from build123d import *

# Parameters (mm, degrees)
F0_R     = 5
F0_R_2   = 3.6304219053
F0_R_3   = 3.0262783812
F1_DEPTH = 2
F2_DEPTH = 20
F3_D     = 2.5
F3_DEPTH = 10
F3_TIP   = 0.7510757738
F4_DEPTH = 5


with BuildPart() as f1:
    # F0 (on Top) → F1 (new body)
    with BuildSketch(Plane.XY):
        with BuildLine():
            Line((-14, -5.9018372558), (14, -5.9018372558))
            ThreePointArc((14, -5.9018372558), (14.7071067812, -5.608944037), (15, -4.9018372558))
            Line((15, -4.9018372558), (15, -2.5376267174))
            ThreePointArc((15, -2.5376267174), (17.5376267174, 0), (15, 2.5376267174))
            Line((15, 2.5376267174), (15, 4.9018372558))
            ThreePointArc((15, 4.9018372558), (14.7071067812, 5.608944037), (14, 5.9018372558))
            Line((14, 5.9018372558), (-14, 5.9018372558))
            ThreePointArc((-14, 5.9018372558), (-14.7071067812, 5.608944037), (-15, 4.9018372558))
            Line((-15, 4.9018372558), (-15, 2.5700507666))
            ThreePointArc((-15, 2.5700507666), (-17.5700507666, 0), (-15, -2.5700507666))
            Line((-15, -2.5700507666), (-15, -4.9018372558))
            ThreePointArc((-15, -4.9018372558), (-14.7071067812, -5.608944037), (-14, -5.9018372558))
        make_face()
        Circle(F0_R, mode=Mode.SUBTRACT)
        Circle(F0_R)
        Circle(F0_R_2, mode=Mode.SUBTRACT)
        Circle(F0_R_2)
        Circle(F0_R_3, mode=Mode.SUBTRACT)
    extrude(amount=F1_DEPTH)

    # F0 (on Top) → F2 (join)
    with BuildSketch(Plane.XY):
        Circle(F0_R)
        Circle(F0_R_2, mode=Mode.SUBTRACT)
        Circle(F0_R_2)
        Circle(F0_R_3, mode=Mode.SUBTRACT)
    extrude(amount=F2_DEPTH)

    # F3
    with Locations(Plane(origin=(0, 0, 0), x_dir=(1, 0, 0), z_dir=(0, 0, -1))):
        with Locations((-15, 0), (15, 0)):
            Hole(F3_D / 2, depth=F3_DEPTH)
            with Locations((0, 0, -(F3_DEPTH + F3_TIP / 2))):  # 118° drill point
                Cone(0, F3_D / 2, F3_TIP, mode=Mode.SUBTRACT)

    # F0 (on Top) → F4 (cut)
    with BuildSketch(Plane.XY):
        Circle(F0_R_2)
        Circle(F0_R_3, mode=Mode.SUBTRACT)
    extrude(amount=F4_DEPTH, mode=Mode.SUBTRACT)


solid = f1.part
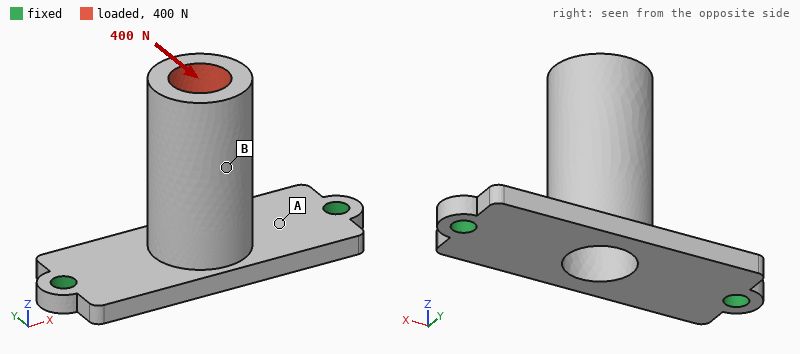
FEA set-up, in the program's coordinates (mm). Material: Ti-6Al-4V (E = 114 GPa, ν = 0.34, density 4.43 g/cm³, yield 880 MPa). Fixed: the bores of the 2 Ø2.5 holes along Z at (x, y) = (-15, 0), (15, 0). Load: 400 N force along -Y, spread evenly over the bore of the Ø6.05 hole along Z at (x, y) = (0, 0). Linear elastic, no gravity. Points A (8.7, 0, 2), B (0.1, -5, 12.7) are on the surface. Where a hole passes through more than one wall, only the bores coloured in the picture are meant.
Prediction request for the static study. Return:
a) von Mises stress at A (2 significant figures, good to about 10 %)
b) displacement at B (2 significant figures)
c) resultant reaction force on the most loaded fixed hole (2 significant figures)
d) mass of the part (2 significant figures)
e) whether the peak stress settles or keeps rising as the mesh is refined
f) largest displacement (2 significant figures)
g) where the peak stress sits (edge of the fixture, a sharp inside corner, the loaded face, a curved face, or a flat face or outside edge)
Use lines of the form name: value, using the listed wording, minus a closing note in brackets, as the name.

von Mises stress at A: 290 MPa
displacement at B: 0.29 mm
resultant reaction force on the most loaded fixed hole: 200 N
mass of the part: 6.7 g
whether the peak stress settles or keeps rising as the mesh is refined: keeps rising
largest displacement: 0.44 mm
where the peak stress sits: edge of the fixture
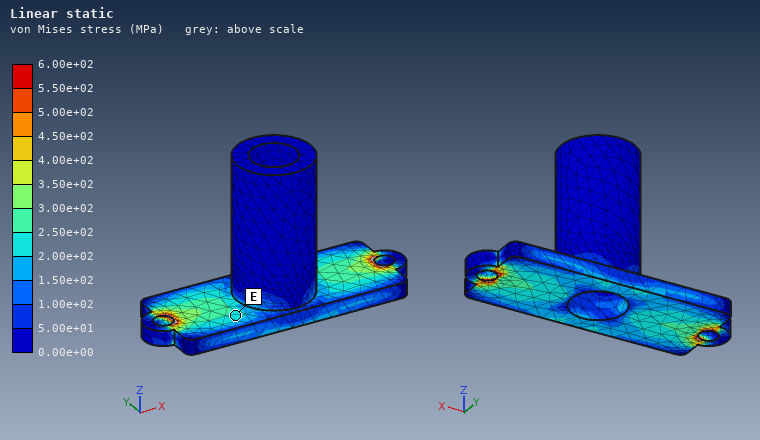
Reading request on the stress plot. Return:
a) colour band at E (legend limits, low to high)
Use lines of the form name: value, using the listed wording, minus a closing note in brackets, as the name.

colour band at E: 2.00e+02 to 2.50e+02 MPa
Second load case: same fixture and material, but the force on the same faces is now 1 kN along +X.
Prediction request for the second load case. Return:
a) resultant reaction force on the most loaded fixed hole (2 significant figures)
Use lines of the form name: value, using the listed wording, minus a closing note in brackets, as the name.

resultant reaction force on the most loaded fixed hole: 740 N
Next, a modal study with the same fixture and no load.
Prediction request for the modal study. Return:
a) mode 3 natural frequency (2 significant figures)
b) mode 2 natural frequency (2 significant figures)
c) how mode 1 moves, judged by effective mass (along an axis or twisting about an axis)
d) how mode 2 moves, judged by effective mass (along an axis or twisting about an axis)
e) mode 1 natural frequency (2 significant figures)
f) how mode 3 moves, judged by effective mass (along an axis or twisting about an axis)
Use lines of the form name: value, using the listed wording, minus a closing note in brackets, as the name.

mode 3 natural frequency: 7100 Hz
mode 2 natural frequency: 6500 Hz
how mode 1 moves, judged by effective mass: along Y
how mode 2 moves, judged by effective mass: along X
mode 1 natural frequency: 3100 Hz
how mode 3 moves, judged by effective mass: along Z
